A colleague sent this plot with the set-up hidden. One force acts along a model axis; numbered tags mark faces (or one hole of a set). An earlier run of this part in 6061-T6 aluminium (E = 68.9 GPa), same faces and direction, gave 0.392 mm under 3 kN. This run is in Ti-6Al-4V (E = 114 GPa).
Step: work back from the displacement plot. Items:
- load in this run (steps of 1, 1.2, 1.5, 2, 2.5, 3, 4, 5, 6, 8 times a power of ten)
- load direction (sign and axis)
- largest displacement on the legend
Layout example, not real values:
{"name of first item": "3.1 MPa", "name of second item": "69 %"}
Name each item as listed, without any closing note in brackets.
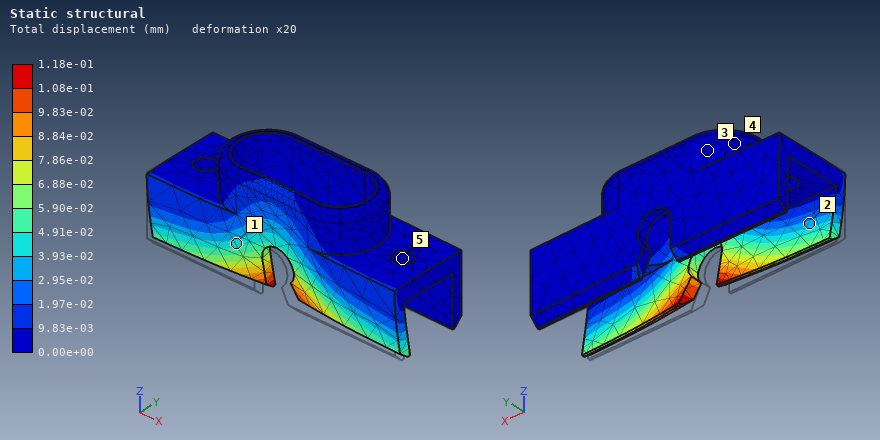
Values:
{"load in this run": "1.5 kN", "load direction": "+Y", "largest displacement on the legend": "1.18e-01 mm"}
